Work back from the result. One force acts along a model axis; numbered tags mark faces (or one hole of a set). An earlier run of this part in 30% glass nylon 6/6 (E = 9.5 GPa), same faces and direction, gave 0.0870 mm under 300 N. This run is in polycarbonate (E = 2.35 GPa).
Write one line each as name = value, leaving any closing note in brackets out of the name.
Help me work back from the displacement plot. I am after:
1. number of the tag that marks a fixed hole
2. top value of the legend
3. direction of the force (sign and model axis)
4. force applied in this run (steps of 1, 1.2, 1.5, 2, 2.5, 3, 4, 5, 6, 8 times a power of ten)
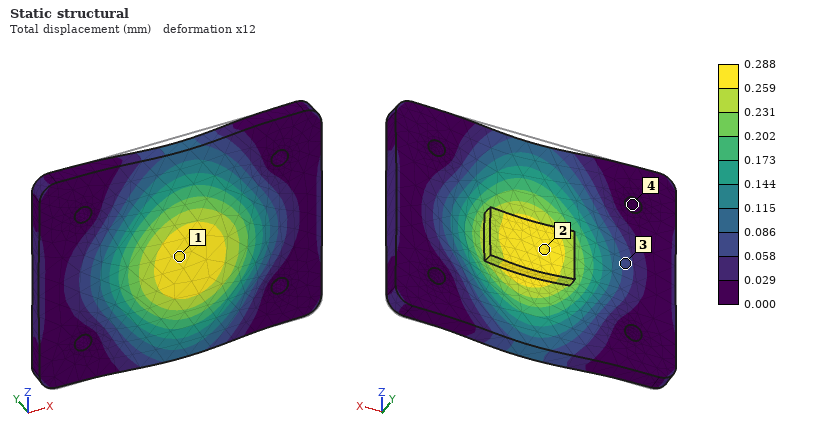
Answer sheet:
number of the tag that marks a fixed hole = 4
top value of the legend = 0.288 mm
direction of the force = -Y
force applied in this run = 250 N
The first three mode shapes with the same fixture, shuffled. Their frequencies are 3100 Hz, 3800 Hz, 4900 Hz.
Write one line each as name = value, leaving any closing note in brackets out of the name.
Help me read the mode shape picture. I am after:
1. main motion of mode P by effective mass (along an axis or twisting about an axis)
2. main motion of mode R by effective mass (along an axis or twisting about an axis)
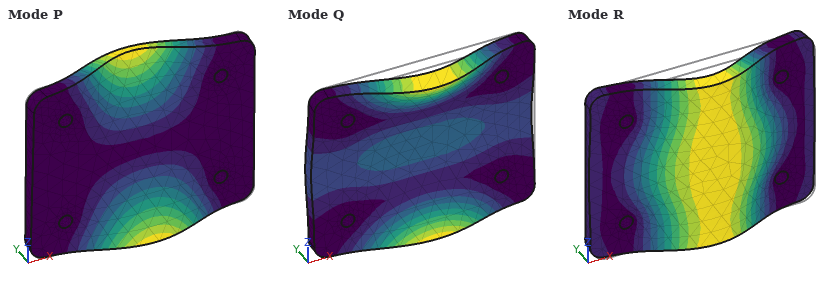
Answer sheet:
main motion of mode P by effective mass = twisting about X
main motion of mode R by effective mass = along Y
